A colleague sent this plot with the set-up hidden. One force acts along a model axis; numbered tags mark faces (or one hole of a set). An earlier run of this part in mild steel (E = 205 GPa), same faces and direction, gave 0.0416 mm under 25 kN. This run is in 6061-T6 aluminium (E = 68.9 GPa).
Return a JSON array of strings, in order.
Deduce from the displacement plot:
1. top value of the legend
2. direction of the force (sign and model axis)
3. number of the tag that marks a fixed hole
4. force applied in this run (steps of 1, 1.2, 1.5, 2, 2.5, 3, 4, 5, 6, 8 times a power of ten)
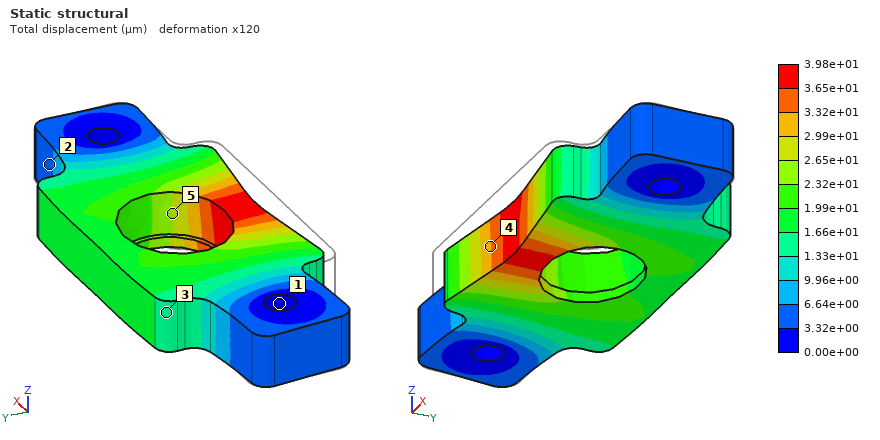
["3.98e+01 µm", "+Y", "1", "8 kN"]
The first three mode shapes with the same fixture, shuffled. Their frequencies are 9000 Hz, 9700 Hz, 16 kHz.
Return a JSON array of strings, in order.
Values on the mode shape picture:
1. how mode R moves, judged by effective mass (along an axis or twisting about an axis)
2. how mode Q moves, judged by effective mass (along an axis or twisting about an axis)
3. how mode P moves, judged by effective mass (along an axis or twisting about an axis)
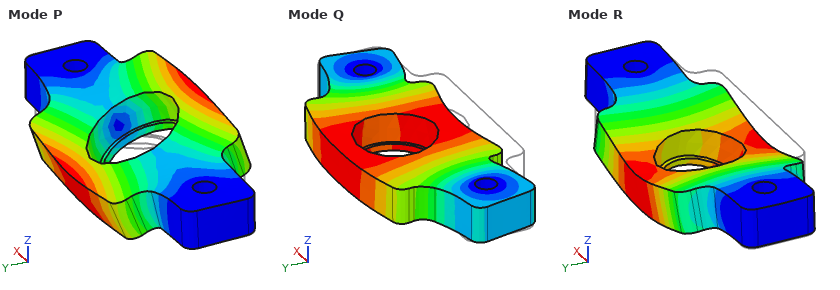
["along Z", "along Y", "twisting about X"]
